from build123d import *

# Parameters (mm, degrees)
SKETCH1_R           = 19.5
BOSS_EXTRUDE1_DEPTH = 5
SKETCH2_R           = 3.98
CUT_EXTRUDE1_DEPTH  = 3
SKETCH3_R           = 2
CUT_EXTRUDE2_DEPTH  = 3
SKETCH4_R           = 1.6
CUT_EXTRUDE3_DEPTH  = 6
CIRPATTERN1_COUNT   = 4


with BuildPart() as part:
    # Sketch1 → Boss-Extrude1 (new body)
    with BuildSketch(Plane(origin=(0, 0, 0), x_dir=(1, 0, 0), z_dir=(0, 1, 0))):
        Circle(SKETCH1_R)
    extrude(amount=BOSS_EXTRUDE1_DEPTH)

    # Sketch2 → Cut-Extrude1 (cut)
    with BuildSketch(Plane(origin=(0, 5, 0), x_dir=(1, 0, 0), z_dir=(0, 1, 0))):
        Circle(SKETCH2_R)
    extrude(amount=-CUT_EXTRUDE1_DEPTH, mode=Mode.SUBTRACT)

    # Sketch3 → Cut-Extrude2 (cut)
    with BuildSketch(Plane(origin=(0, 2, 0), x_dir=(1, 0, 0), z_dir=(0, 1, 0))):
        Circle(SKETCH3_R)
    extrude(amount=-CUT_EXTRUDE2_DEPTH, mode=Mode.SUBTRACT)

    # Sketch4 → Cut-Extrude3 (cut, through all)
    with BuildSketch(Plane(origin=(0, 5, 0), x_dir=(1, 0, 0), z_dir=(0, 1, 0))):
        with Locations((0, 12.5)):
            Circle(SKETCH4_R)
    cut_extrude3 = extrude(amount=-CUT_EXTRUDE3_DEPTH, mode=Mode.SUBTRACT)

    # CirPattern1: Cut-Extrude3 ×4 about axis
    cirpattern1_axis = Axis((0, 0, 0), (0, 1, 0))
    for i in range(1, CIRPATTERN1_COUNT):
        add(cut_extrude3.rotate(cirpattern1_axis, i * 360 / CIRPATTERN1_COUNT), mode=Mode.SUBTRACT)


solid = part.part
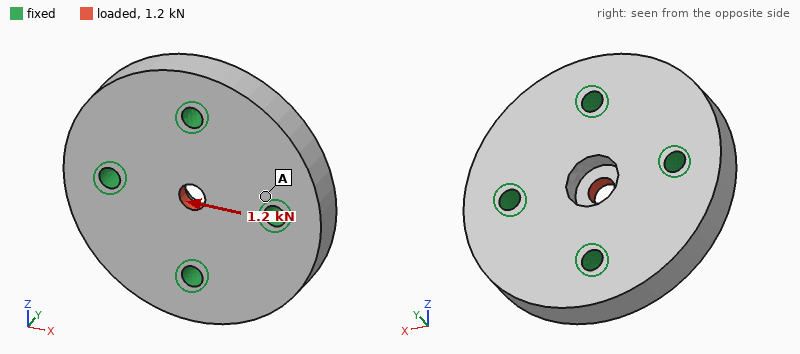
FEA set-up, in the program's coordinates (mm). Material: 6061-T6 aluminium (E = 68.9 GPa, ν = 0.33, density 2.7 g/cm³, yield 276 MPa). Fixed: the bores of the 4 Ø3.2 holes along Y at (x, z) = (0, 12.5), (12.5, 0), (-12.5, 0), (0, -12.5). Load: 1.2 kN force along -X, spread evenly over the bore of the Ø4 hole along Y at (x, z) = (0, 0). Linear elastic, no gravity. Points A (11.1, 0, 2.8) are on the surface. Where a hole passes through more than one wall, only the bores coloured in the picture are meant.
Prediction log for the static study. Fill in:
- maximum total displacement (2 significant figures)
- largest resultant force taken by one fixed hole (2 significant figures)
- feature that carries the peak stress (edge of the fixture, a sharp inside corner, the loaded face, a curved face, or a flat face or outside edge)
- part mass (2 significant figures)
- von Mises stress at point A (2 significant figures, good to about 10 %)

3.8 µm
410 N
the loaded face
15 g
6.8 MPa
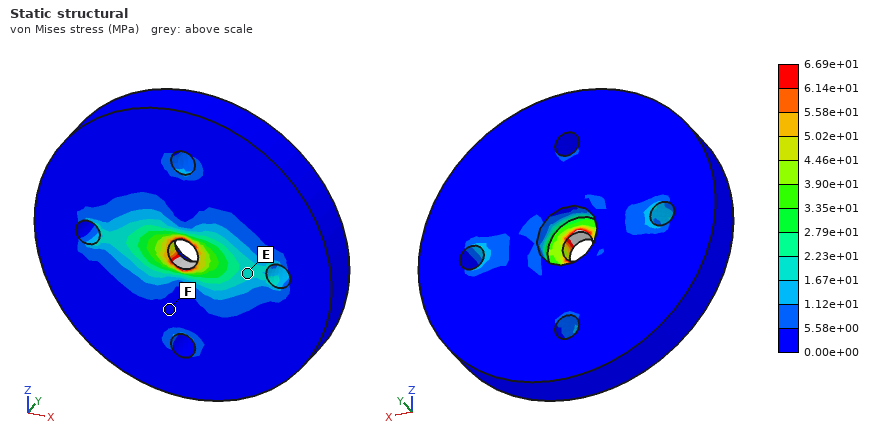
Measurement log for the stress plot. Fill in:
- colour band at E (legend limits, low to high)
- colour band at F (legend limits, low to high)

1.67e+01 to 2.23e+01 MPa
0.00e+00 to 5.58e+00 MPa
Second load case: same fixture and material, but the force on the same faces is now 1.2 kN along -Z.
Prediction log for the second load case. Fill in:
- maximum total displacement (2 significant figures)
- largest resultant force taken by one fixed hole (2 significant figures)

3.8 µm
410 N
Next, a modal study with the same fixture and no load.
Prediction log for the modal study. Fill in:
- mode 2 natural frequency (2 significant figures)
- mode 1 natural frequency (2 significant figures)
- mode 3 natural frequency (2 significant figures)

34 kHz
32 kHz
34 kHz
